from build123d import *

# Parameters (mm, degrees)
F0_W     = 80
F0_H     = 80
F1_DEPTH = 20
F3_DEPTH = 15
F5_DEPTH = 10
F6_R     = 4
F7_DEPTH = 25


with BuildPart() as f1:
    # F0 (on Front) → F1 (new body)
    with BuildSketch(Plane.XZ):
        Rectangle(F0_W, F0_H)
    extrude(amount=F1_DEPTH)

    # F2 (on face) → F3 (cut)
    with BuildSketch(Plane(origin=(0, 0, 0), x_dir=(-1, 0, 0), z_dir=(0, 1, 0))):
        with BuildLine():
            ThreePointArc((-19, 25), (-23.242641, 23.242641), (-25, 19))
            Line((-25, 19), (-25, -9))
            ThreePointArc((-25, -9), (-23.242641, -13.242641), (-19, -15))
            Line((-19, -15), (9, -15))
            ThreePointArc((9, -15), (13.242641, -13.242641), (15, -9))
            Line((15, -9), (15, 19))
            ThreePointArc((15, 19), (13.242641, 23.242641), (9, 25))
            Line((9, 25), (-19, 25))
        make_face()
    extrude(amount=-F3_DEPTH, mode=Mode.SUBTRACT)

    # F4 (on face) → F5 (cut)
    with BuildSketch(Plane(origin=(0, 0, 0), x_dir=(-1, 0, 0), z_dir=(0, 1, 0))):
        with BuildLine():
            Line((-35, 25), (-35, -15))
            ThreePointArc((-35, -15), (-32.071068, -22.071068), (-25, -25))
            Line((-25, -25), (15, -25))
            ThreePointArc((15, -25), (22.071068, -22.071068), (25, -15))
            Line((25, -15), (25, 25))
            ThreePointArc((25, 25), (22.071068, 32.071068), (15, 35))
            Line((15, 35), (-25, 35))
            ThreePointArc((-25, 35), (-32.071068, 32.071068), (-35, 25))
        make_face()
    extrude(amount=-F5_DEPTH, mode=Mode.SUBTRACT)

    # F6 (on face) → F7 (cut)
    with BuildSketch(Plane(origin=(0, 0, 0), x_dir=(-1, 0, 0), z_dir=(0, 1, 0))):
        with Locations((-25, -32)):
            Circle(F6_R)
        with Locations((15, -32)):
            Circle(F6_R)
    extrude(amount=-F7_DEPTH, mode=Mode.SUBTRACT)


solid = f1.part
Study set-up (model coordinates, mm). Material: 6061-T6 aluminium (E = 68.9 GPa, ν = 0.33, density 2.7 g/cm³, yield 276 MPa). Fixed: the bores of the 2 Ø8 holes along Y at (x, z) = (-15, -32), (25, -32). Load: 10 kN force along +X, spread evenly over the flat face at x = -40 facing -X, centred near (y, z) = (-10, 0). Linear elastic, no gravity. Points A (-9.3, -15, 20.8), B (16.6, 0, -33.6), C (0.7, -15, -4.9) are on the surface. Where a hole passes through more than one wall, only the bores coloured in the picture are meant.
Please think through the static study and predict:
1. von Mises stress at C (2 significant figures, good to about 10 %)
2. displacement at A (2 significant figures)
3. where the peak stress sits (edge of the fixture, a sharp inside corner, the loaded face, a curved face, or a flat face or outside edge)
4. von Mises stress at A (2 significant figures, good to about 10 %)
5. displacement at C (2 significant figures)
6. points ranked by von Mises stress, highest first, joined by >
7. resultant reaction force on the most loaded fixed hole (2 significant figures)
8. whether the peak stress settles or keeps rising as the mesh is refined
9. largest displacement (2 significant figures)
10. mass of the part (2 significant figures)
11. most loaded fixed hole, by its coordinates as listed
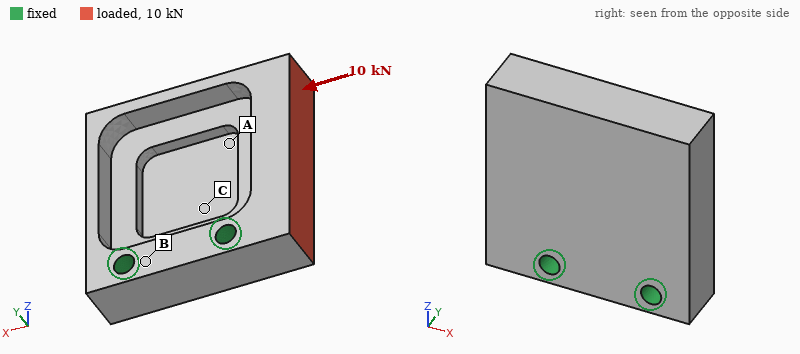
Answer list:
42 MPa
0.054 mm
edge of the fixture
28 MPa
0.023 mm
C > A > B
9.0 kN
keeps rising
0.13 mm
220 g
(-15, -32)
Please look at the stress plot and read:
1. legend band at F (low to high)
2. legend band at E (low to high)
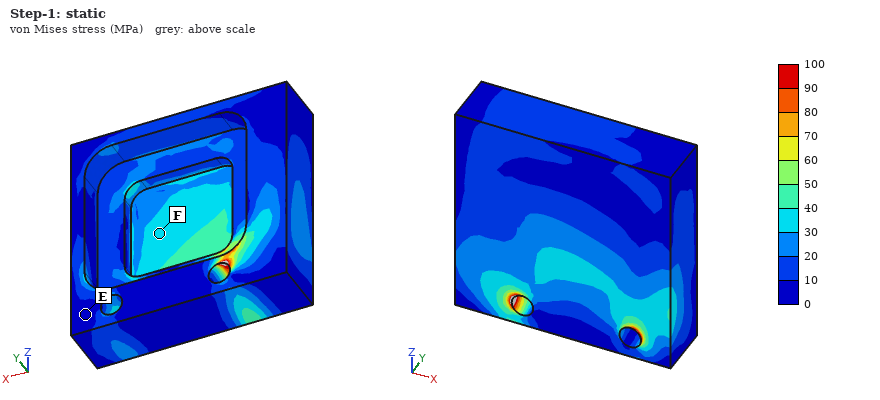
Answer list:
30 to 40 MPa
0 to 10 MPa
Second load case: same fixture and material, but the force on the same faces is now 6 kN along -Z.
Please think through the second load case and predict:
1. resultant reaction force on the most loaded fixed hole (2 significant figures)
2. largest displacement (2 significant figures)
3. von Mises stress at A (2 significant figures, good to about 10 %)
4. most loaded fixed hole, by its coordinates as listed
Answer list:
8.4 kN
56 µm
7.8 MPa
(-15, -32)
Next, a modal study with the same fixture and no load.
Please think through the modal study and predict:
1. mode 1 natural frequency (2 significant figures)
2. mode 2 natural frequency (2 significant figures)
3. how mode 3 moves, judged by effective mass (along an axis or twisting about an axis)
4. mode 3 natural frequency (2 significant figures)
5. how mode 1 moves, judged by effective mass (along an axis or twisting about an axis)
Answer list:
2100 Hz
3100 Hz
along X
5400 Hz
along Y
